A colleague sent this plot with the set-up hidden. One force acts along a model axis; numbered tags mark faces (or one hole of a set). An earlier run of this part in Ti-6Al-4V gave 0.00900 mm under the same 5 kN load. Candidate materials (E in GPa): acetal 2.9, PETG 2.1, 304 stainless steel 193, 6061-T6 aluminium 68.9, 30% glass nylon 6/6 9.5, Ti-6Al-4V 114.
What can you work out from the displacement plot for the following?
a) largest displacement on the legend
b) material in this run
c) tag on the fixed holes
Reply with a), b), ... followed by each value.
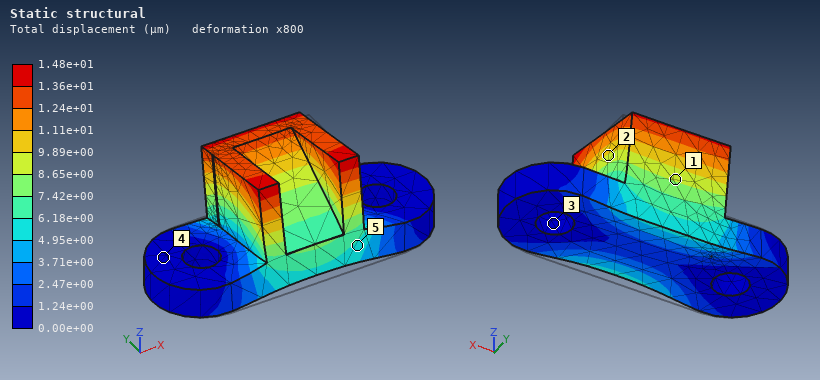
a) 1.48e+01 µm
b) 6061-T6 aluminium
c) 3
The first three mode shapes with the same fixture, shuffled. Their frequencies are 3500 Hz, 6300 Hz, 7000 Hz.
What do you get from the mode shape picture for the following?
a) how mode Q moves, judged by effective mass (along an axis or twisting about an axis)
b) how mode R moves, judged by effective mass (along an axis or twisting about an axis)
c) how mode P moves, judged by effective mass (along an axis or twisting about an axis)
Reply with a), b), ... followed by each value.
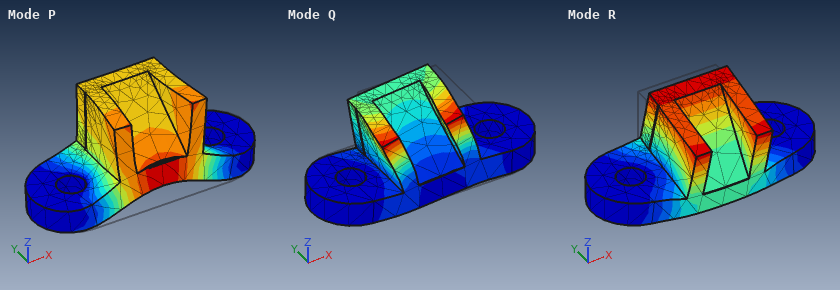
a) along X
b) along Y
c) along Z
